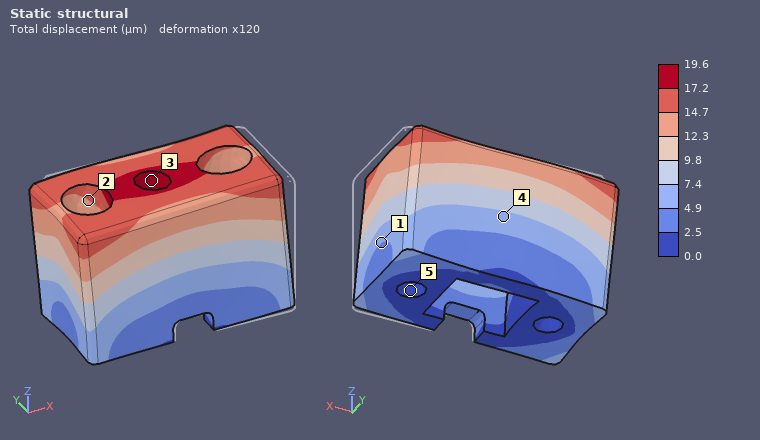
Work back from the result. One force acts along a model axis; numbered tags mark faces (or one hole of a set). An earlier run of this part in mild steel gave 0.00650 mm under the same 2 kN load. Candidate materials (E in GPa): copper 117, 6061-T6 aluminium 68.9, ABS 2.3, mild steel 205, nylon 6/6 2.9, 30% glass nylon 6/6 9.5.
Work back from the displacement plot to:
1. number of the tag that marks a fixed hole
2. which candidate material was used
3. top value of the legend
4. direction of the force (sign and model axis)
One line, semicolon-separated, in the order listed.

5; 6061-T6 aluminium; 19.6 µm; -X
